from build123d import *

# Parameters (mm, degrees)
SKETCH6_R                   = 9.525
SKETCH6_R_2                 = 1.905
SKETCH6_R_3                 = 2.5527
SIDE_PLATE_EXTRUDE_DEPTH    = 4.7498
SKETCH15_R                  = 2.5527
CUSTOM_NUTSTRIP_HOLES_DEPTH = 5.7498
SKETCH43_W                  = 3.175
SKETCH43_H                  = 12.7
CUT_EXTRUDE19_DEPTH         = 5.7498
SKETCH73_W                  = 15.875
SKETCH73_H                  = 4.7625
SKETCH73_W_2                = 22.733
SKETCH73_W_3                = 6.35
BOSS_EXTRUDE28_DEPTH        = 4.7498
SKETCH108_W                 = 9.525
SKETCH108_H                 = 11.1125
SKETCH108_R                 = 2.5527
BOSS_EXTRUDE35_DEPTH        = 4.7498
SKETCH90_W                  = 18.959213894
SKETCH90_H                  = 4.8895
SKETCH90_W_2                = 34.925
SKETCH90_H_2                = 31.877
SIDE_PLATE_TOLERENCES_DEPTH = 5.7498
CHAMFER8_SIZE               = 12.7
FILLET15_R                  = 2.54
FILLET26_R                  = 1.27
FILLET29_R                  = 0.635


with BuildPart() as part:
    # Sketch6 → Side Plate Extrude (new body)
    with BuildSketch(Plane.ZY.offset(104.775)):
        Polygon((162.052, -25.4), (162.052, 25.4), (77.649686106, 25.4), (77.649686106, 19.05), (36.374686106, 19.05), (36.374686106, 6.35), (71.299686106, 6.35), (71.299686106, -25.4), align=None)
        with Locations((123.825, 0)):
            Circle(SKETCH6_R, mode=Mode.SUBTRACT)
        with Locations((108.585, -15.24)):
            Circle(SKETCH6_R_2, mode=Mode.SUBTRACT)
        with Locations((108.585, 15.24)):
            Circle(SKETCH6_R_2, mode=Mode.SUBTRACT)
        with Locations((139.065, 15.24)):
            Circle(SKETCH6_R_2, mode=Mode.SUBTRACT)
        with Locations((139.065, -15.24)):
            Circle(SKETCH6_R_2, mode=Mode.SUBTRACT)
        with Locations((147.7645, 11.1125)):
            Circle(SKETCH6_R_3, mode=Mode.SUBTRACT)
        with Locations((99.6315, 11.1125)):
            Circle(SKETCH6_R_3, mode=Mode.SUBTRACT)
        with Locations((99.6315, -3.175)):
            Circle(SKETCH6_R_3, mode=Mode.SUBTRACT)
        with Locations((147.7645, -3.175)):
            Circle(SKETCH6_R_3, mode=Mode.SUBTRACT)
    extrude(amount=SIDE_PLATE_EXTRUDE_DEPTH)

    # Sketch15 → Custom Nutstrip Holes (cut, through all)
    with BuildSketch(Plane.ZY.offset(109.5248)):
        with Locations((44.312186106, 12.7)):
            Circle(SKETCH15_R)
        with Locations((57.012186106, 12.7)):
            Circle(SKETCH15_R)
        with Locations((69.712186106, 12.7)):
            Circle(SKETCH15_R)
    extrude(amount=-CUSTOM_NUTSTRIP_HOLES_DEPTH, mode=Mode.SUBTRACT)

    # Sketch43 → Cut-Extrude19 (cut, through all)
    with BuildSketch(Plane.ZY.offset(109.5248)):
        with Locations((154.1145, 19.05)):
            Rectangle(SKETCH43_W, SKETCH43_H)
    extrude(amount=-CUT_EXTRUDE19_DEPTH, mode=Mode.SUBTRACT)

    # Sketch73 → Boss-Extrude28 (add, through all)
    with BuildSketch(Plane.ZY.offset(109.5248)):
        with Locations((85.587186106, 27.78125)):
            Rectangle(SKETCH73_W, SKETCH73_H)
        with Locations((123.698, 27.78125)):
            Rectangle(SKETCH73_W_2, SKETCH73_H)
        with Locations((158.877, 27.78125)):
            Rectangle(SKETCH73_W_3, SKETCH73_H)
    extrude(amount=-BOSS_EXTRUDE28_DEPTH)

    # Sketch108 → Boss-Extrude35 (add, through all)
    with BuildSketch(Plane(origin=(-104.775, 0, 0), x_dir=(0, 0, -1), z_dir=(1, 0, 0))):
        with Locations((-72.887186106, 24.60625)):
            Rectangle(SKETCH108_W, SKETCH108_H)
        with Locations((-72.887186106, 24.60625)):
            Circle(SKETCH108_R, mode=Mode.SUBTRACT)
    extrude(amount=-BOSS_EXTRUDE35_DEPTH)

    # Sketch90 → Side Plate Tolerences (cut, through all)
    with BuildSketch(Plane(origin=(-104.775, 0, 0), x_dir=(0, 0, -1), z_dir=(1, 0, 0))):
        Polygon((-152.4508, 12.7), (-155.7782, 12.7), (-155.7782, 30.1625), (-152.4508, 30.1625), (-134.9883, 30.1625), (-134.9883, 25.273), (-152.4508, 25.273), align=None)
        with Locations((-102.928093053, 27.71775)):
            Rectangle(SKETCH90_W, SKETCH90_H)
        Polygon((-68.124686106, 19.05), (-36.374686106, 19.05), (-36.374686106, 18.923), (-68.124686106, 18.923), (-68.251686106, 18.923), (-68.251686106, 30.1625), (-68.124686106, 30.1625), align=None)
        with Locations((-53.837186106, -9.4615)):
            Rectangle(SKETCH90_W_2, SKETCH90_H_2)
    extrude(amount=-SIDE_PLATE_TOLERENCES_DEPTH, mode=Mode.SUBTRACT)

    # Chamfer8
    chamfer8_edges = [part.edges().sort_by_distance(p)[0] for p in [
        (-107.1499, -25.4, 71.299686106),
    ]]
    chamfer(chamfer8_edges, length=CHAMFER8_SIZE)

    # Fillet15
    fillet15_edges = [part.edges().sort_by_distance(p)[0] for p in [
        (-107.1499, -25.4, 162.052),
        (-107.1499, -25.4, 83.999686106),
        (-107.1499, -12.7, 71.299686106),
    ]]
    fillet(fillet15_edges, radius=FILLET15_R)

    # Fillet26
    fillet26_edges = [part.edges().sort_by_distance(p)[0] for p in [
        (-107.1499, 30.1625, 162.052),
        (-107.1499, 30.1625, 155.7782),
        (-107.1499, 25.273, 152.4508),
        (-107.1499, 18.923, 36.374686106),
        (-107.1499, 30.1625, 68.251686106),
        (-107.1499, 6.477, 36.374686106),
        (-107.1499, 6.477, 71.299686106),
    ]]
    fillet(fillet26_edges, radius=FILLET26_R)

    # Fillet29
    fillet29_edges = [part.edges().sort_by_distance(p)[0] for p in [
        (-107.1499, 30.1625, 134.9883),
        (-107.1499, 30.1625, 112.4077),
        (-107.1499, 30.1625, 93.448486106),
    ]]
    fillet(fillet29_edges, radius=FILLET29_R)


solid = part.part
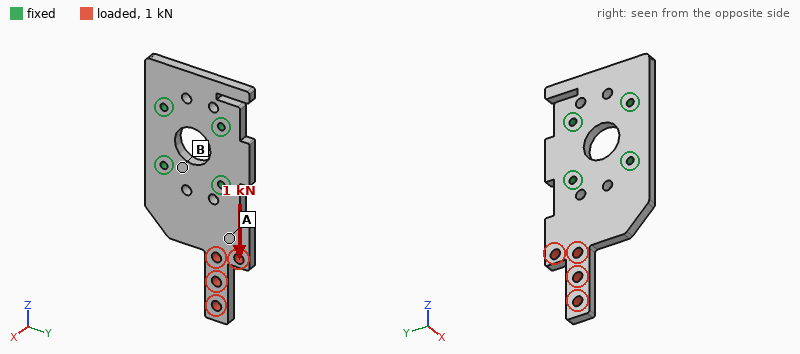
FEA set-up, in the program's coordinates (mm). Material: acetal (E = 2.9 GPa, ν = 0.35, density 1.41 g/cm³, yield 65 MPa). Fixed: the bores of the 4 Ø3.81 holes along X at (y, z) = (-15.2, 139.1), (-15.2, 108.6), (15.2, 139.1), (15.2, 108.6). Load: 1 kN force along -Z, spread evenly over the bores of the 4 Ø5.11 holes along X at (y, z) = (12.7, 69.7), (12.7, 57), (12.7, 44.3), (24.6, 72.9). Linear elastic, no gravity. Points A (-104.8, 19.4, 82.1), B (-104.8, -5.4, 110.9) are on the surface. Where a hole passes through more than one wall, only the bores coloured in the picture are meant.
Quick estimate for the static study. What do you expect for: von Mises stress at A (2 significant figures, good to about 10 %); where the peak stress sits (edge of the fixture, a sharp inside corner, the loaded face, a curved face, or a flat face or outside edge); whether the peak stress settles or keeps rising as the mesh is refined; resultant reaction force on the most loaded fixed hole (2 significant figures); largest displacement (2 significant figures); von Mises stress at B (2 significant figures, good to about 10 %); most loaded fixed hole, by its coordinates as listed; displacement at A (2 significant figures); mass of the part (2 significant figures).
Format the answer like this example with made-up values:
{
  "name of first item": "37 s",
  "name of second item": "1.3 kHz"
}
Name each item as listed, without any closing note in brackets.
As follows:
{
  "von Mises stress at A": "10 MPa",
  "where the peak stress sits": "edge of the fixture",
  "whether the peak stress settles or keeps rising as the mesh is refined": "keeps rising",
  "resultant reaction force on the most loaded fixed hole": "820 N",
  "largest displacement": "0.33 mm",
  "von Mises stress at B": "2.3 MPa",
  "most loaded fixed hole, by its coordinates as listed": "(15.2, 108.6)",
  "displacement at A": "0.14 mm",
  "mass of the part": "31 g"
}
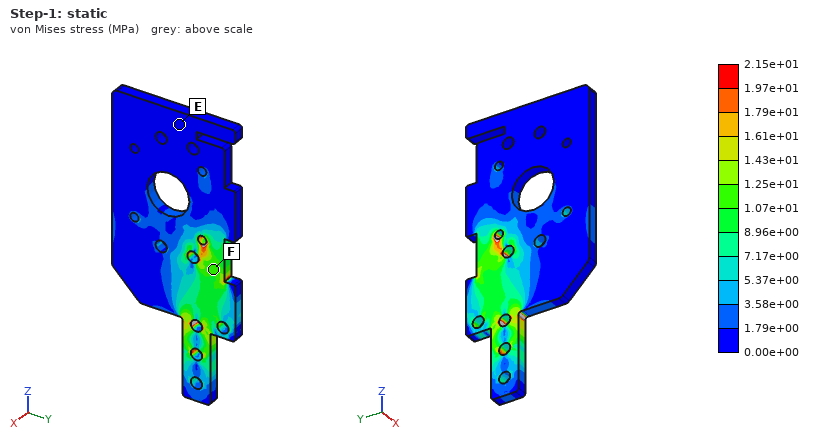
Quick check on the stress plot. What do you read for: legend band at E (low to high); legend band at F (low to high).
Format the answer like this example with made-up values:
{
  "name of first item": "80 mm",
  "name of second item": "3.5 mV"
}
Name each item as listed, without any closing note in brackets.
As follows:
{
  "legend band at E": "0.00e+00 to 1.79e+00 MPa",
  "legend band at F": "1.07e+01 to 1.25e+01 MPa"
}
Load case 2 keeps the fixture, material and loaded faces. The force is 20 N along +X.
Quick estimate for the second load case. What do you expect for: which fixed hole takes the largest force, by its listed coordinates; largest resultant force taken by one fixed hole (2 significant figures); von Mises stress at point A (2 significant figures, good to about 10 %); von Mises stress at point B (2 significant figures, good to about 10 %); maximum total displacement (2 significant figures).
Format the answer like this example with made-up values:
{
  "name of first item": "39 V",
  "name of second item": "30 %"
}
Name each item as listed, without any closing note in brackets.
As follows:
{
  "which fixed hole takes the largest force, by its listed coordinates": "(15.2, 108.6)",
  "largest resultant force taken by one fixed hole": "23 N",
  "von Mises stress at point A": "2.8 MPa",
  "von Mises stress at point B": "1.8 MPa",
  "maximum total displacement": "1.6 mm"
}
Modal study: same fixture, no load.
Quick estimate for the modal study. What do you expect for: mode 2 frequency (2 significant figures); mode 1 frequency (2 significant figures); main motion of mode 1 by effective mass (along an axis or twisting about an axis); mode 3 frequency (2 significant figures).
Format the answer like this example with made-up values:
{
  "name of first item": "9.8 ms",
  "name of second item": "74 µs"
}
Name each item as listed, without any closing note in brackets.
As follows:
{
  "mode 2 frequency": "1100 Hz",
  "mode 1 frequency": "340 Hz",
  "main motion of mode 1 by effective mass": "along X",
  "mode 3 frequency": "1400 Hz"
}
